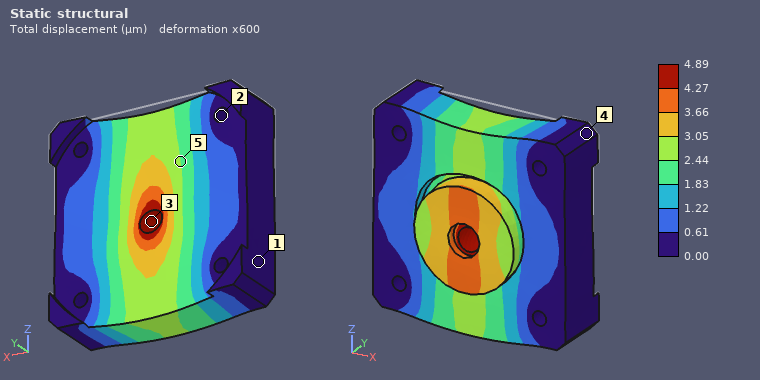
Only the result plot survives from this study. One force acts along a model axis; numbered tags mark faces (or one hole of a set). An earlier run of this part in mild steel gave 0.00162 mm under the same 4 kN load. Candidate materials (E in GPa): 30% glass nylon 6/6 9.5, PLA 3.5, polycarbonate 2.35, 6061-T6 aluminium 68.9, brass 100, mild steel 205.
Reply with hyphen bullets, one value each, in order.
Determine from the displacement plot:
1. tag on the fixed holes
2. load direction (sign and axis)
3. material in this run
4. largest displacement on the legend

- 2
- -Z
- 6061-T6 aluminium
- 4.89 µm
